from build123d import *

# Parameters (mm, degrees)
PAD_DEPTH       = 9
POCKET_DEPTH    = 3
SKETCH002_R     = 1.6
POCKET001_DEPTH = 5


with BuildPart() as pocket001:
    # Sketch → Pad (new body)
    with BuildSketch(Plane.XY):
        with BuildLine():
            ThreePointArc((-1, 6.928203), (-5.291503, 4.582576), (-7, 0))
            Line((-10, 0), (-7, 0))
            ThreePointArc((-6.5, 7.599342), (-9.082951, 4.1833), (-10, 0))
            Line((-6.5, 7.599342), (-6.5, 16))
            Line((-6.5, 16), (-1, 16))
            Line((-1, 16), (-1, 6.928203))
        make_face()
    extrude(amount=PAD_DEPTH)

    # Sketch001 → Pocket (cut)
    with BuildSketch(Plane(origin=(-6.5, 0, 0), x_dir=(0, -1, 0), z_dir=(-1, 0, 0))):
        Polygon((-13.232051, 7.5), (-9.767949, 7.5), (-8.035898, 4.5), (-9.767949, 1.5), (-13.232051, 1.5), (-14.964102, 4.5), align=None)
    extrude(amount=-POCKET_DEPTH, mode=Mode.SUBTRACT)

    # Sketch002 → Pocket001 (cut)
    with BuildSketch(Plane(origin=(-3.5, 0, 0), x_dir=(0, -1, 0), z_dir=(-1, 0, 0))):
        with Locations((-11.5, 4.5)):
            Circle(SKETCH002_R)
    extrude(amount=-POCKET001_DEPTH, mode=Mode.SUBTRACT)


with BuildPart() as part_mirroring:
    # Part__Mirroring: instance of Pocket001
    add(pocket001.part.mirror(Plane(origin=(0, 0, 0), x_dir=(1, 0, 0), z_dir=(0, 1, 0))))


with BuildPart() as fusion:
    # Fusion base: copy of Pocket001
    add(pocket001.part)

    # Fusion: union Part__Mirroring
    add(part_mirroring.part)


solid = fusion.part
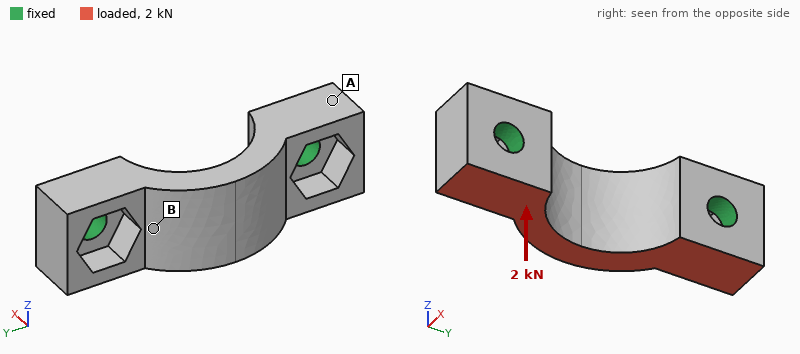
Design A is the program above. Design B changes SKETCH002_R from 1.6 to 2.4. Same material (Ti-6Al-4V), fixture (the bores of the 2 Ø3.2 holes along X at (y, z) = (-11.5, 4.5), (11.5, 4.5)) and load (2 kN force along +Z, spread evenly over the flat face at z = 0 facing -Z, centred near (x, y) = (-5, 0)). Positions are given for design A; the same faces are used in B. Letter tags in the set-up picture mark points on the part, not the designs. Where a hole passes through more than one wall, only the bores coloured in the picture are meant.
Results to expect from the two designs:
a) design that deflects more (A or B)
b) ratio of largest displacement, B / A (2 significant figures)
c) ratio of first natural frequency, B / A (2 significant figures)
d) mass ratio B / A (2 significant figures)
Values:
A
0.58
1.3
0.96
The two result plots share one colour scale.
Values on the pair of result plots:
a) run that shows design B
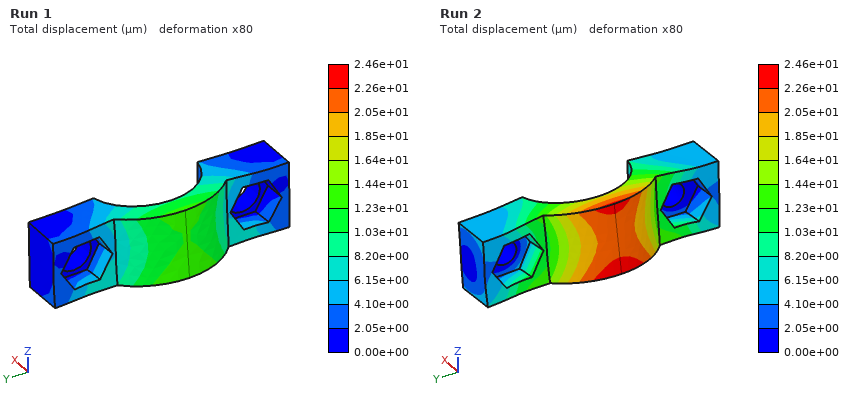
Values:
Run 1
